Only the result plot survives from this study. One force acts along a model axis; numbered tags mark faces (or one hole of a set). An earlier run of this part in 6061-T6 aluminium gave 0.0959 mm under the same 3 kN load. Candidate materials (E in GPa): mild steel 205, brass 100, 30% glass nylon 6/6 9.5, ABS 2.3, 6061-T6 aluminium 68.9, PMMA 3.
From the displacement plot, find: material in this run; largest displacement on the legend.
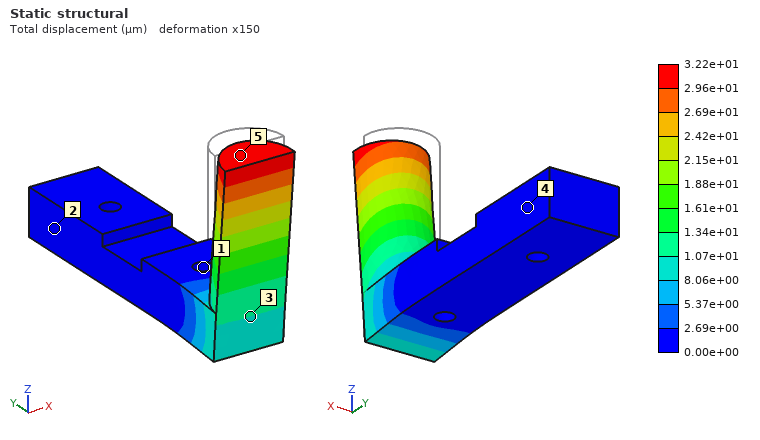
mild steel
3.22e+01 µm
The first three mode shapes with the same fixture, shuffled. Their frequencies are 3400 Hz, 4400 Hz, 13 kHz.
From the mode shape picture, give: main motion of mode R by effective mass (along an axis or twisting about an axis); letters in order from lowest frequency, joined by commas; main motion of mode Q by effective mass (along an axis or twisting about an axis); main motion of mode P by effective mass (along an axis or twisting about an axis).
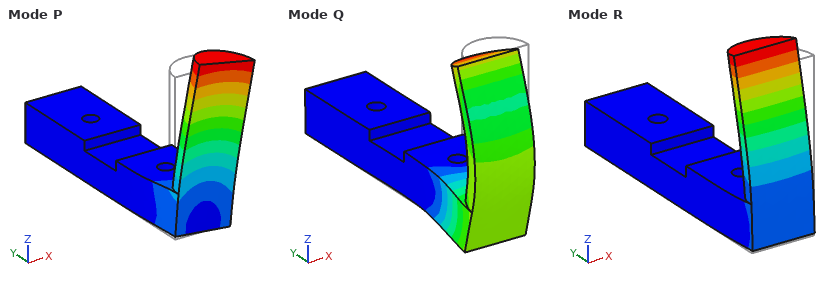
along Y
R, P, Q
along Z
along X
